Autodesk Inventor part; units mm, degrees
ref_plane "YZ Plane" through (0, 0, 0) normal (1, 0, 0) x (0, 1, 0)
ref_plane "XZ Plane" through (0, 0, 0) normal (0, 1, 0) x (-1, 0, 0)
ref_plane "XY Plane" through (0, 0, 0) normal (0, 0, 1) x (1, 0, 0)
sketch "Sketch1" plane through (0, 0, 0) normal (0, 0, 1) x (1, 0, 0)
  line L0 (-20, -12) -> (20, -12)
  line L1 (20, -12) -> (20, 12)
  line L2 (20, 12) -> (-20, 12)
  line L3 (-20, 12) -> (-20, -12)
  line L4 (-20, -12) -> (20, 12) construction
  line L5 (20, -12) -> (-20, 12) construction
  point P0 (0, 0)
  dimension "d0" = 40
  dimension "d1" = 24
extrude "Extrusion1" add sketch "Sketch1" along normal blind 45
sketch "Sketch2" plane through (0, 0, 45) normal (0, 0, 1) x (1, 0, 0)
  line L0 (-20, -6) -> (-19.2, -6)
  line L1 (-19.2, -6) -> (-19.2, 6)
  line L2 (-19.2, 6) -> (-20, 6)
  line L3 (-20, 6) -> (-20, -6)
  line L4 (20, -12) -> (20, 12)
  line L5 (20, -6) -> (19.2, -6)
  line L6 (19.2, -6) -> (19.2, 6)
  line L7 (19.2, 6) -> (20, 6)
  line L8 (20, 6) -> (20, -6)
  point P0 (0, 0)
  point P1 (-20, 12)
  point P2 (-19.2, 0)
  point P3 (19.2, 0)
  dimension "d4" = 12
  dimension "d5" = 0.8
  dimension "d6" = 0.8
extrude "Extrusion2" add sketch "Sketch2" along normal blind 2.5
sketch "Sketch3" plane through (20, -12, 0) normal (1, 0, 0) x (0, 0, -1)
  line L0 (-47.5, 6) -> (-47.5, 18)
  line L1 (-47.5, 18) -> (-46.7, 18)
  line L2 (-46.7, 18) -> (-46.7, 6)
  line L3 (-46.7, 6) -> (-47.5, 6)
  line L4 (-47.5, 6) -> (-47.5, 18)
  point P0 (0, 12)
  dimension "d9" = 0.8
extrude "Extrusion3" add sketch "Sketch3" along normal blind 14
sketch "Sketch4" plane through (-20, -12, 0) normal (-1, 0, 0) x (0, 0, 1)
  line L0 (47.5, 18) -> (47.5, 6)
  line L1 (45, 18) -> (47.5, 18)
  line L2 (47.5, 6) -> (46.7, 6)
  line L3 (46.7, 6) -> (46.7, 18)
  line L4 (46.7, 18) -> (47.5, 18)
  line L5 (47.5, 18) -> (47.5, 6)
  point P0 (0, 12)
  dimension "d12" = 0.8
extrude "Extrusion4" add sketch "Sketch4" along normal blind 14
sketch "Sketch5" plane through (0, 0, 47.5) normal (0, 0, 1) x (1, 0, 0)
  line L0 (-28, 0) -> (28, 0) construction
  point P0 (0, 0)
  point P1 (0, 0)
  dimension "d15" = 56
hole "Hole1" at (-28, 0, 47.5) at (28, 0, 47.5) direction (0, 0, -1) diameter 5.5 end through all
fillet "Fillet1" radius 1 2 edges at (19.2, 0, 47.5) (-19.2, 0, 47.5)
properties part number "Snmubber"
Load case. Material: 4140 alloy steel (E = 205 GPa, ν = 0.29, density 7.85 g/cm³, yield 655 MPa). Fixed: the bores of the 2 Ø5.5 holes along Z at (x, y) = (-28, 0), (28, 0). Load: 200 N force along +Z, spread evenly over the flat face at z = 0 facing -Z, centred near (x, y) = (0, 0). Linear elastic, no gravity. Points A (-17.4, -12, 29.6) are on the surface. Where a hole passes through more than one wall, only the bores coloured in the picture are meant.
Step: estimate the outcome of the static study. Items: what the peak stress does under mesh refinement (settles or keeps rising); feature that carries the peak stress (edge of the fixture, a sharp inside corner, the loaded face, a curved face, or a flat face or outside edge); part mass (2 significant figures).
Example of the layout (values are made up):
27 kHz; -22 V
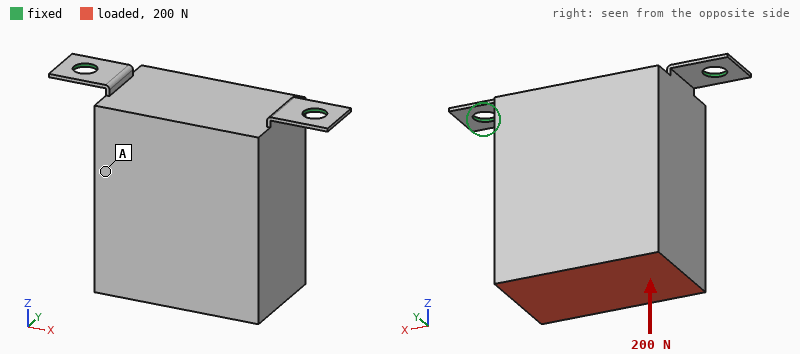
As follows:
keeps rising; edge of the fixture; 340 g
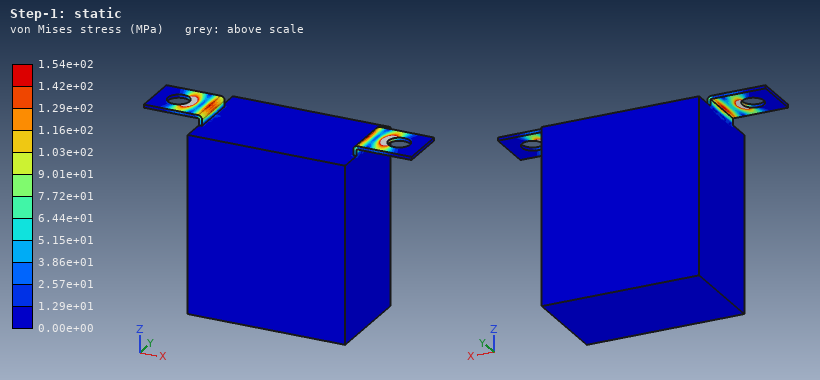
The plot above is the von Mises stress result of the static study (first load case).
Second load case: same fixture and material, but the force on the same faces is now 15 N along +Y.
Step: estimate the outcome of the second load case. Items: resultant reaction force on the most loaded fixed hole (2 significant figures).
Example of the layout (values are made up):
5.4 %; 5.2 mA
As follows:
7.5 N
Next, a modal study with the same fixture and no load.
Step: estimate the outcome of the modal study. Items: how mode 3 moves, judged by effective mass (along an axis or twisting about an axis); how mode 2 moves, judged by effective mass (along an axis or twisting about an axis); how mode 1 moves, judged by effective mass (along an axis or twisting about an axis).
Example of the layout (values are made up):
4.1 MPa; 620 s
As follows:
along Z; along X; along Y
